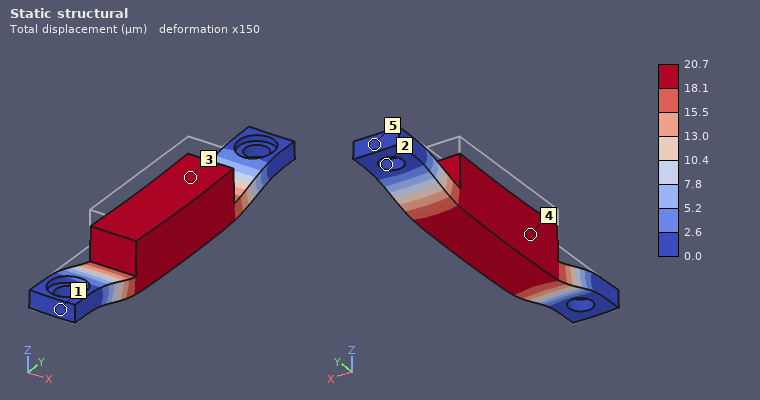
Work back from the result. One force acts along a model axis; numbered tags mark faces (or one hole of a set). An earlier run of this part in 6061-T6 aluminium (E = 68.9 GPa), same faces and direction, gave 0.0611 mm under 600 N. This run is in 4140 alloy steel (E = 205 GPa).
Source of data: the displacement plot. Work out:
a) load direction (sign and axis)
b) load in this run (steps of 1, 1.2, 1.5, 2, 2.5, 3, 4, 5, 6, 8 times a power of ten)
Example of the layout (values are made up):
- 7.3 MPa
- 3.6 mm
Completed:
- -Z
- 600 N
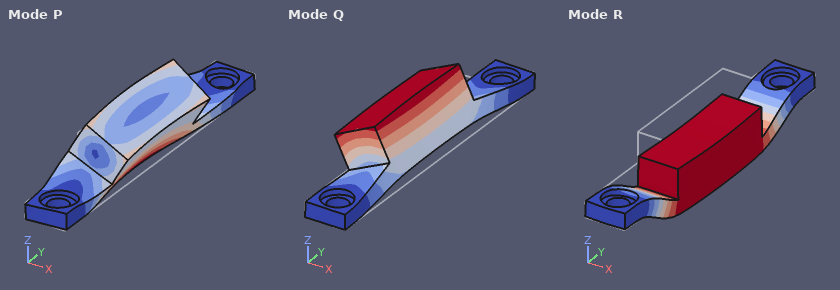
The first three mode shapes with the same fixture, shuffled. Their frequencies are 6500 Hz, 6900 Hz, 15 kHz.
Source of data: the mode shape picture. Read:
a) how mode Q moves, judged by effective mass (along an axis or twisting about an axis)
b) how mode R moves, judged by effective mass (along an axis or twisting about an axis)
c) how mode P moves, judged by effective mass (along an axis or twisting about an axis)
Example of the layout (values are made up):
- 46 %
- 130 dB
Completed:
- along X
- along Z
- along X
